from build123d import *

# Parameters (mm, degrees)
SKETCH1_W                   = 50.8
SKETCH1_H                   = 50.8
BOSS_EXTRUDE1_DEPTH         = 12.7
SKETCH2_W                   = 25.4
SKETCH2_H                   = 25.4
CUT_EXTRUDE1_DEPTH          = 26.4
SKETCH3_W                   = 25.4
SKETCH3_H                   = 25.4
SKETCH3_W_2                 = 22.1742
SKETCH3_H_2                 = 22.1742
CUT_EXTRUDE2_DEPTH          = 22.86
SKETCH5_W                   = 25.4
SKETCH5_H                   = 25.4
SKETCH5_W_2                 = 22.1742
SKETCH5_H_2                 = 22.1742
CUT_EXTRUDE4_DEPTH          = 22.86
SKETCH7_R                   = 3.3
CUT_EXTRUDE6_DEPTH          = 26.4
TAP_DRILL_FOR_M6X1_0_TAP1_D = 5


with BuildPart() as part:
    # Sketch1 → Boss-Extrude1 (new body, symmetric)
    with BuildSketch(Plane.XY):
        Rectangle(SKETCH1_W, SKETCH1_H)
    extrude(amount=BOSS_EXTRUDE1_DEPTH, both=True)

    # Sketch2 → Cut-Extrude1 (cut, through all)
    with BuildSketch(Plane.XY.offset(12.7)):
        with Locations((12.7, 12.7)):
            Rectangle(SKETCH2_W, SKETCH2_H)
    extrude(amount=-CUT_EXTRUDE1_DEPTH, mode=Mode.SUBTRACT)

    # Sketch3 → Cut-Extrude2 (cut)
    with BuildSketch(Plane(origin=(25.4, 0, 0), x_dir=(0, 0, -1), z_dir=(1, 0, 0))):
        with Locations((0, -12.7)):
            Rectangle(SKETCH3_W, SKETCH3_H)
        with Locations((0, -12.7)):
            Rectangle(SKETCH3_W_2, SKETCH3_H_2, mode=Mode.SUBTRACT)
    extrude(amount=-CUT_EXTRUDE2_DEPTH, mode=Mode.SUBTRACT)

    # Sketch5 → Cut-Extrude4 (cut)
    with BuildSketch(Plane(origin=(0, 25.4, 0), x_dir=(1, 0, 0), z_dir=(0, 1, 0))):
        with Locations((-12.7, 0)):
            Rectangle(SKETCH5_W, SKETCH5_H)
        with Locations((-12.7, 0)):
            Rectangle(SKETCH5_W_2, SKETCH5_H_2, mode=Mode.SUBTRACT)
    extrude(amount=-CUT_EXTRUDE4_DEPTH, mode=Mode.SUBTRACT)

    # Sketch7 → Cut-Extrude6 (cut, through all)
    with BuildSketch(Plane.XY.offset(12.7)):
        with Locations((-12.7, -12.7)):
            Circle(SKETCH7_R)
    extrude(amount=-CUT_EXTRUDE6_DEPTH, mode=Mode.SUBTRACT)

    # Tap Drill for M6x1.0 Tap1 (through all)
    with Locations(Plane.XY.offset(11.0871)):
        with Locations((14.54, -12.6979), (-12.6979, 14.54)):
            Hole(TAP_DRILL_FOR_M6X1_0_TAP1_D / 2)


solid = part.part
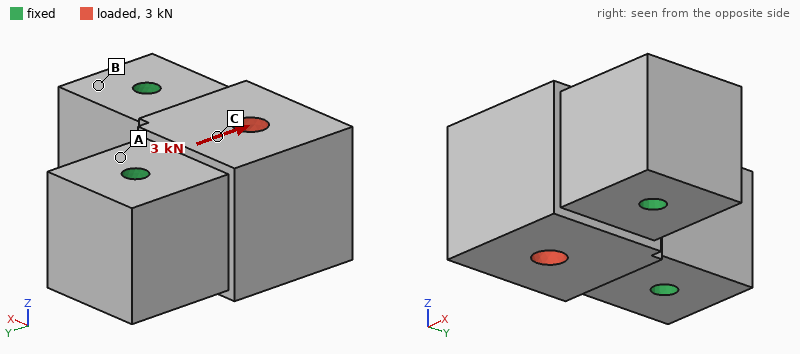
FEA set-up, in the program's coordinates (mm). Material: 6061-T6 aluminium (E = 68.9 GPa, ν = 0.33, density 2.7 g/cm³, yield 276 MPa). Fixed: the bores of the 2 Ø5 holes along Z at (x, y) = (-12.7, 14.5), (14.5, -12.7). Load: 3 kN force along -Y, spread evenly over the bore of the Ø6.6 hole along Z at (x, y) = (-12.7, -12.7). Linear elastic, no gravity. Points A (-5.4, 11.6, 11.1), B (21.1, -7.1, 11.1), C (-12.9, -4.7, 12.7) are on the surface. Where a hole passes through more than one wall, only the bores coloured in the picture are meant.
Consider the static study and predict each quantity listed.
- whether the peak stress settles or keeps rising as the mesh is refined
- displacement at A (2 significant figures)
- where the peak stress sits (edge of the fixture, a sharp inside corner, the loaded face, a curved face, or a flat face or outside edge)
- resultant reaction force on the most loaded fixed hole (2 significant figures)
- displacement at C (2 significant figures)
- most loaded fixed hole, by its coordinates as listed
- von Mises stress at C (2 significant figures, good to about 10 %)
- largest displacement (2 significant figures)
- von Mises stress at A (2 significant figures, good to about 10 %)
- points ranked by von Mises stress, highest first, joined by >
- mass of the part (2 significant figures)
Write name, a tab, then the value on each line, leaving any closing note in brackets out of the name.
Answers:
whether the peak stress settles or keeps rising as the mesh is refined	keeps rising
displacement at A	0.75 µm
where the peak stress sits	edge of the fixture
resultant reaction force on the most loaded fixed hole	2.7 kN
displacement at C	1.9 µm
most loaded fixed hole, by its coordinates as listed	(-12.7, 14.5)
von Mises stress at C	6.3 MPa
largest displacement	3.2 µm
von Mises stress at A	2.7 MPa
points ranked by von Mises stress, highest first, joined by >	C > A > B
mass of the part	110 g
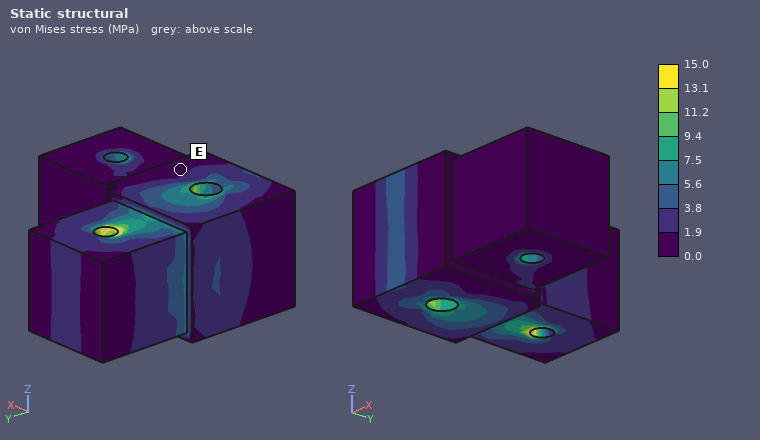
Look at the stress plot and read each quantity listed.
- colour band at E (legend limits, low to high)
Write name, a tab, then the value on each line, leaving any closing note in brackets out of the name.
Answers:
colour band at E	0.0 to 1.9 MPa
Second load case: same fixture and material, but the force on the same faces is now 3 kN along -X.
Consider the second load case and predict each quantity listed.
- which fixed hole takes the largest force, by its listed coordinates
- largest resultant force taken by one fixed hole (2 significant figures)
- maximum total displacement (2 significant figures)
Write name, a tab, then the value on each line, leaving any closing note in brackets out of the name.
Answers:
which fixed hole takes the largest force, by its listed coordinates	(14.5, -12.7)
largest resultant force taken by one fixed hole	2.7 kN
maximum total displacement	3.2 µm
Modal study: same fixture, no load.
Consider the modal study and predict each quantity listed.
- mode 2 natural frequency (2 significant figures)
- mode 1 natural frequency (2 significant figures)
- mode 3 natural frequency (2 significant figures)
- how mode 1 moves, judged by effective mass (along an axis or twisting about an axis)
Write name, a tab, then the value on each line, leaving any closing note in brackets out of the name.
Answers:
mode 2 natural frequency	24 kHz
mode 1 natural frequency	12 kHz
mode 3 natural frequency	28 kHz
how mode 1 moves, judged by effective mass	along Z
